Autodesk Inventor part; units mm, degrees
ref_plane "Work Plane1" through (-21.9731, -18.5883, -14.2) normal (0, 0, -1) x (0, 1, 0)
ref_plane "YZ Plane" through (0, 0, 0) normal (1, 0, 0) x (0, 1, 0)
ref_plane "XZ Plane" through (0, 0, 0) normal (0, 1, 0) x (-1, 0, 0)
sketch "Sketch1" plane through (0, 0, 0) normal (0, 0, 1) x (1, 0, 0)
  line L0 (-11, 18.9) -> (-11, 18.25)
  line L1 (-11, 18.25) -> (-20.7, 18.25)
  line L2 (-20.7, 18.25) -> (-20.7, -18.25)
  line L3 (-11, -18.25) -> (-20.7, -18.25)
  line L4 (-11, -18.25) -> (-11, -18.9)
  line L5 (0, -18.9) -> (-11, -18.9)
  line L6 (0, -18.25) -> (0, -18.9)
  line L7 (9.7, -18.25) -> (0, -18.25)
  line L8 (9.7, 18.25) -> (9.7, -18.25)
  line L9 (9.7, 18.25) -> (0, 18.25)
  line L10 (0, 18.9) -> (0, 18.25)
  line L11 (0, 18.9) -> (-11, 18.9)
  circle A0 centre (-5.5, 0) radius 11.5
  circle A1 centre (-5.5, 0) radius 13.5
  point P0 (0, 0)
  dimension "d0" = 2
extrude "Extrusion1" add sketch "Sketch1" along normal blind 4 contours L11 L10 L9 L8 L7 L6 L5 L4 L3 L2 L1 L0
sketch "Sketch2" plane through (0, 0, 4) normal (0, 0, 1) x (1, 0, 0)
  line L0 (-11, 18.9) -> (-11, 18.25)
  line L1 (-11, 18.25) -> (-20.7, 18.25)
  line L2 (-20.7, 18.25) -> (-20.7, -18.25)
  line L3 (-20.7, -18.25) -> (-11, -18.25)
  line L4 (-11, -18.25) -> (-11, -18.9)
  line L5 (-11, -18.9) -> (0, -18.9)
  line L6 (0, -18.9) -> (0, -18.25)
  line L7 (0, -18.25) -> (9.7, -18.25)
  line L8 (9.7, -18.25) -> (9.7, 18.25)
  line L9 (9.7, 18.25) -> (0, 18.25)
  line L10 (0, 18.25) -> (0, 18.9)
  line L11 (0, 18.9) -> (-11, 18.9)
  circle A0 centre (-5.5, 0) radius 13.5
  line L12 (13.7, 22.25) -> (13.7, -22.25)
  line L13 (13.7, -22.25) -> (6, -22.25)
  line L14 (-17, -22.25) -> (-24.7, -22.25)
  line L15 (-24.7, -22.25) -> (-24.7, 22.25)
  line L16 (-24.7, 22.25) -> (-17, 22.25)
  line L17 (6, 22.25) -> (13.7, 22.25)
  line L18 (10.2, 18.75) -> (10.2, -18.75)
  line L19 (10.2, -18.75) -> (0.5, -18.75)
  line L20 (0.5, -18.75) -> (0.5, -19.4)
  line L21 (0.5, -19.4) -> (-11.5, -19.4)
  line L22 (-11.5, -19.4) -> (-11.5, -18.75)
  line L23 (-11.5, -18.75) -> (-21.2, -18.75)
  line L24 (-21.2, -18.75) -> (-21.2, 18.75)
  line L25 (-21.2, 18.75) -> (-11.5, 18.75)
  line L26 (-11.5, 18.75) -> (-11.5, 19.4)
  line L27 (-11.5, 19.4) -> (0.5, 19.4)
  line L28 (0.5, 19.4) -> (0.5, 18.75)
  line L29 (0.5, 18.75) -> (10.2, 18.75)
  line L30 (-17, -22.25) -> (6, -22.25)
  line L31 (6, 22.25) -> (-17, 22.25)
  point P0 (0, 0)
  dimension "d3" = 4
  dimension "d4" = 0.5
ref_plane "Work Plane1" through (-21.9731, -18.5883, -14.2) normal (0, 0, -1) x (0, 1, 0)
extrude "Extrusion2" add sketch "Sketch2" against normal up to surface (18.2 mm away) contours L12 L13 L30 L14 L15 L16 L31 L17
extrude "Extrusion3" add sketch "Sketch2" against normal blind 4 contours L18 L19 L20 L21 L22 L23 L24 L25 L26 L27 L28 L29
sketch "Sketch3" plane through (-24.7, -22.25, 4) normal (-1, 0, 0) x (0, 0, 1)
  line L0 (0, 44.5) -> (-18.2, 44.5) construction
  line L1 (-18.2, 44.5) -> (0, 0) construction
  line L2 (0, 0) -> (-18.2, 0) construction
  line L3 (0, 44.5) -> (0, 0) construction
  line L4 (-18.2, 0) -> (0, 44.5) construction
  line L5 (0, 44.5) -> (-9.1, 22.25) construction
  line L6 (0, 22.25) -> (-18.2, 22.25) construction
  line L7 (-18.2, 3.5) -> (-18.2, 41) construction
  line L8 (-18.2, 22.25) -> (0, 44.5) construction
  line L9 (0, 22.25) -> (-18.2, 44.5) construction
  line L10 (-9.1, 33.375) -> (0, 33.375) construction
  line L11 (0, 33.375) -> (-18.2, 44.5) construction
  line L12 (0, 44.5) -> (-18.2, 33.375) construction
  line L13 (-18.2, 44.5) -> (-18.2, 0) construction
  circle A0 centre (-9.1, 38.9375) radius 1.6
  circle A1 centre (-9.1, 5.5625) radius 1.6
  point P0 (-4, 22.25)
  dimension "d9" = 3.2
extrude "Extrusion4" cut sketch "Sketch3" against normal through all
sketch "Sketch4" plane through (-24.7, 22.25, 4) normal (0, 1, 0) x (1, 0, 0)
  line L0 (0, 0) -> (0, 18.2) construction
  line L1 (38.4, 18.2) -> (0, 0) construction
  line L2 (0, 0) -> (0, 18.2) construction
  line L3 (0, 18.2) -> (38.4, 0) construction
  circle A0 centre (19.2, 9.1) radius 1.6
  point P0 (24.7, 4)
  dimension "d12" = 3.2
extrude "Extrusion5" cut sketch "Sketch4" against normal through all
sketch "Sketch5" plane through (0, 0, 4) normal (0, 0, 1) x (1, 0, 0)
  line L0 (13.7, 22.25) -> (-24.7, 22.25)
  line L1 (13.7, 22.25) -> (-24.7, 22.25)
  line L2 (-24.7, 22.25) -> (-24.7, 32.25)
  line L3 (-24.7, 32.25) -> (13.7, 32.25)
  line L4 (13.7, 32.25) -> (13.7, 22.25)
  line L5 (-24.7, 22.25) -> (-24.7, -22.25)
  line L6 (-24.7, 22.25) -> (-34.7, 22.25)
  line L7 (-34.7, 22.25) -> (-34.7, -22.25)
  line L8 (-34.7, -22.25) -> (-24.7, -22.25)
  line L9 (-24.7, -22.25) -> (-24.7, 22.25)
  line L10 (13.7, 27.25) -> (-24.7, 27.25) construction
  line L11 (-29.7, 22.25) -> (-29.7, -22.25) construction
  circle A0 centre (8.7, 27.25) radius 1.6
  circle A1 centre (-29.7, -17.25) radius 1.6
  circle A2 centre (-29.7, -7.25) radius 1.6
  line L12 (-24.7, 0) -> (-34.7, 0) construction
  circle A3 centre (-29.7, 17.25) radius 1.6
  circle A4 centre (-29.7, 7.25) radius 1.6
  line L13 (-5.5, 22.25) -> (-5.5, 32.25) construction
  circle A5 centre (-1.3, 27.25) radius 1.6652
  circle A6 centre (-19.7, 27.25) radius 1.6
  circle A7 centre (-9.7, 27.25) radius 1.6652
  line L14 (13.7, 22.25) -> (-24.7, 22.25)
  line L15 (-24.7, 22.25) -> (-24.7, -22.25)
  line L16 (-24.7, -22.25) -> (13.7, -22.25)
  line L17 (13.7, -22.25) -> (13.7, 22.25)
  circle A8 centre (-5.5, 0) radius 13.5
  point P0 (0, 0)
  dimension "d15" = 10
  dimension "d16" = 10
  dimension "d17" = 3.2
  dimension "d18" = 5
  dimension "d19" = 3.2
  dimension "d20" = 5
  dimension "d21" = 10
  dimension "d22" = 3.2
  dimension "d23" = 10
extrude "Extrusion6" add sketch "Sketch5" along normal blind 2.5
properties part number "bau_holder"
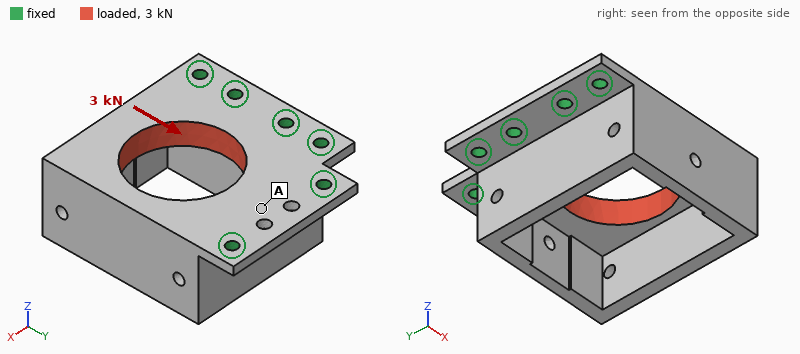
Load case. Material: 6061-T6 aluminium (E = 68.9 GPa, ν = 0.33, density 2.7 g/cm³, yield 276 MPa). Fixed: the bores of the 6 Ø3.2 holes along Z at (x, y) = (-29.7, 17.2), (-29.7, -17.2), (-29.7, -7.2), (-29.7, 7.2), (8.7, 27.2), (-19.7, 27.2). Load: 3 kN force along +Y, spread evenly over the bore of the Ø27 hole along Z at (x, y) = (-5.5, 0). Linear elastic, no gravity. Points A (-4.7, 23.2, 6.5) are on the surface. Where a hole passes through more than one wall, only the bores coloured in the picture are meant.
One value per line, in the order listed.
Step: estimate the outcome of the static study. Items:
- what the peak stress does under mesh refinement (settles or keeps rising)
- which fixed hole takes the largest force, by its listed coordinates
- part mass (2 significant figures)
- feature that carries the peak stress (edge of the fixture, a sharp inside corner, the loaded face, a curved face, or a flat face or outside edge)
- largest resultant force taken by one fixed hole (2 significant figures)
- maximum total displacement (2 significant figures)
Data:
keeps rising
(8.7, 27.2)
44 g
edge of the fixture
1.2 kN
50 µm
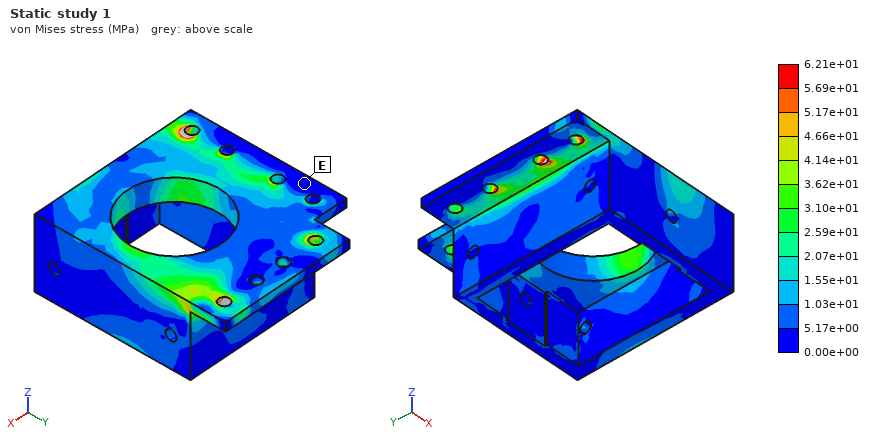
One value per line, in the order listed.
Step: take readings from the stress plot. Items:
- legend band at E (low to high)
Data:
0.00e+00 to 5.17e+00 MPa
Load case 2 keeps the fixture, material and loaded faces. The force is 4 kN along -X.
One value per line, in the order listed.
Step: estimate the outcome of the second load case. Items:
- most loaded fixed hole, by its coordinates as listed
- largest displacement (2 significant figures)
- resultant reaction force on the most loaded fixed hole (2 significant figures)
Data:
(-29.7, -17.2)
90 µm
1.2 kN
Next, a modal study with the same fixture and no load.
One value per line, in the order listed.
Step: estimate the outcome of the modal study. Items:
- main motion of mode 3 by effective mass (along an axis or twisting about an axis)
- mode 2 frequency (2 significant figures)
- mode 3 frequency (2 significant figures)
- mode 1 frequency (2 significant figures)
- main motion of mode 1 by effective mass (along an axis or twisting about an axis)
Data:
along Z
9800 Hz
11 kHz
2000 Hz
along Z
